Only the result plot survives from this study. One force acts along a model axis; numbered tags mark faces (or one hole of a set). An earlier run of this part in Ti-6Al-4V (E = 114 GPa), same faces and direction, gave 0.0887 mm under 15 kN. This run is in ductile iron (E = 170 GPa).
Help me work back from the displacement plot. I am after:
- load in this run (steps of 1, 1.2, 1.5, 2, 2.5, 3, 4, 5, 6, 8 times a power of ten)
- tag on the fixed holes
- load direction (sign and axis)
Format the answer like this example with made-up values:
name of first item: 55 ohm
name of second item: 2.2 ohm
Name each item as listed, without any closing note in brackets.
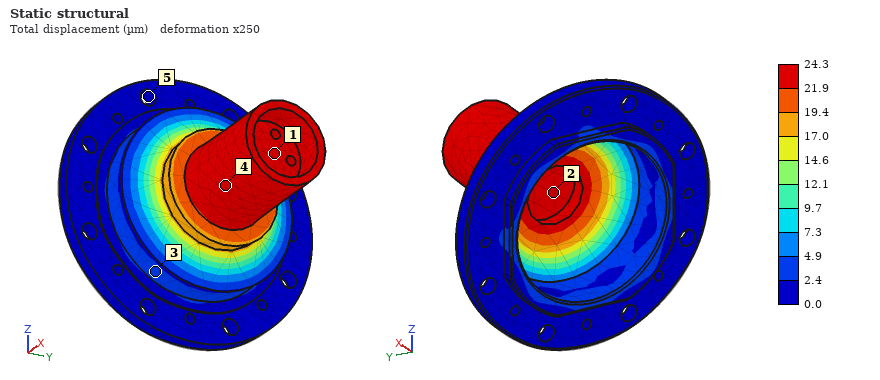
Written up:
load in this run: 6 kN
tag on the fixed holes: 5
load direction: +X
